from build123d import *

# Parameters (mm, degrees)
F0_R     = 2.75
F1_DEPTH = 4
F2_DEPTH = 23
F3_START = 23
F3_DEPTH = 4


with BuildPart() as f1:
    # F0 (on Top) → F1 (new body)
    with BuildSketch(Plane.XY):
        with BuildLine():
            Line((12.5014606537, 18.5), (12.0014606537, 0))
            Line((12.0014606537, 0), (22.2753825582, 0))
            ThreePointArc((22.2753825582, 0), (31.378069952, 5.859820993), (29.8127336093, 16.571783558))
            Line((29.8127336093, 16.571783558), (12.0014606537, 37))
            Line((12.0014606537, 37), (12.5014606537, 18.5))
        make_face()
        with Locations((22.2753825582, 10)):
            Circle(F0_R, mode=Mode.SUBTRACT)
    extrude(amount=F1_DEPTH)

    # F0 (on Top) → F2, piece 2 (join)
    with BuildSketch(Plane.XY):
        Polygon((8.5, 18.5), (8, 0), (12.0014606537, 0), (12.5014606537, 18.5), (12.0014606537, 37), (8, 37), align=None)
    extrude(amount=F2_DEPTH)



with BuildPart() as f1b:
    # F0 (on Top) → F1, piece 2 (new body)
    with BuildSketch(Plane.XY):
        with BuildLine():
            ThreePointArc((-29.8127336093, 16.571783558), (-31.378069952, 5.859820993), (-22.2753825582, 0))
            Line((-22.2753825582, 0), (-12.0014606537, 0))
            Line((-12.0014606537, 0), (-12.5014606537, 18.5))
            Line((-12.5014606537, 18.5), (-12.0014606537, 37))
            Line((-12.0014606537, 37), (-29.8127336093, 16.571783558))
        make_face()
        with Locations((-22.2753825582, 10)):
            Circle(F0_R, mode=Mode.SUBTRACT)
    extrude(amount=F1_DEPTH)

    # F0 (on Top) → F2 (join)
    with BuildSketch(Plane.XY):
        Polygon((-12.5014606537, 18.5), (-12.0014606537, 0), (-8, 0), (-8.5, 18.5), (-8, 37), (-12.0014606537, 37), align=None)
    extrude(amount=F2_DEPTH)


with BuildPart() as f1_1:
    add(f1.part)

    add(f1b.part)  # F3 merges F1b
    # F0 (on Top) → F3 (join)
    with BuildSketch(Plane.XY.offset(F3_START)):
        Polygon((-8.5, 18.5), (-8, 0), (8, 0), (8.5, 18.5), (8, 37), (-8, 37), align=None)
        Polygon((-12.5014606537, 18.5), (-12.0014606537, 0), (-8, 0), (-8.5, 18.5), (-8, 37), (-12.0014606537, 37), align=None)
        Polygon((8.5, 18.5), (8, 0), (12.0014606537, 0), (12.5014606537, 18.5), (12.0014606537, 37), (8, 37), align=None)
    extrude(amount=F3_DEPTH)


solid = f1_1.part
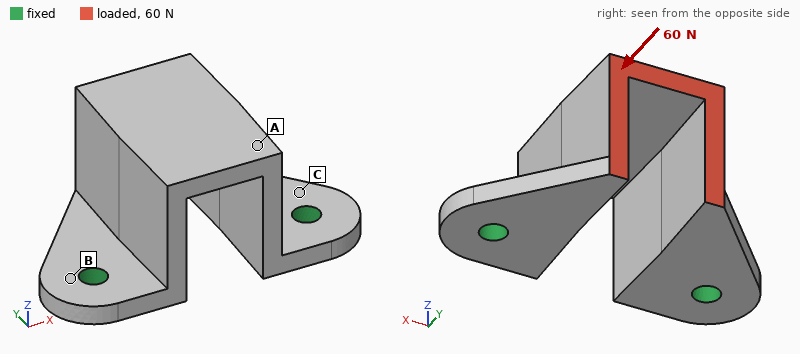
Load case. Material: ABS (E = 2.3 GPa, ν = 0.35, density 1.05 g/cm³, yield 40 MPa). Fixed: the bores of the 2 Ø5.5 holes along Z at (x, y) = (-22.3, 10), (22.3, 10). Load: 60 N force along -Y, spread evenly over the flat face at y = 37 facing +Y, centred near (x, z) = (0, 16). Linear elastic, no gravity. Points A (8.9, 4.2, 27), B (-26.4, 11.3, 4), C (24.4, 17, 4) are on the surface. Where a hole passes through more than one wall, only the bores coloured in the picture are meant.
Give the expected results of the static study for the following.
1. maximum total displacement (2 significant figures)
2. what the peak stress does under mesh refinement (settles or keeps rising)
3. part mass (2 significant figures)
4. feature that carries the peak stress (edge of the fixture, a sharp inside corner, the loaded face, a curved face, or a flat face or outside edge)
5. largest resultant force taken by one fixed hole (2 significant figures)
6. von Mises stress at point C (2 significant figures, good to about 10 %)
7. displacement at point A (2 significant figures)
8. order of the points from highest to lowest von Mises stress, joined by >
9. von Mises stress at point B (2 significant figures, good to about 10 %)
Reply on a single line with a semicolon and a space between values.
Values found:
0.31 mm; keeps rising; 15 g; edge of the fixture; 30 N; 3.0 MPa; 0.23 mm; C > B > A; 1.5 MPa
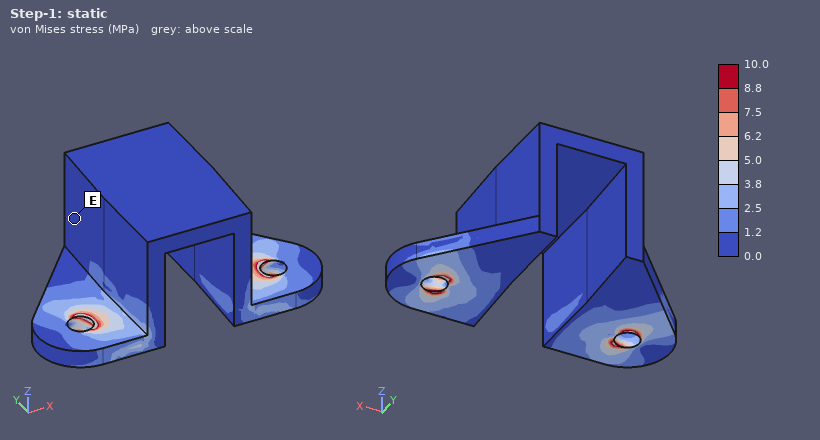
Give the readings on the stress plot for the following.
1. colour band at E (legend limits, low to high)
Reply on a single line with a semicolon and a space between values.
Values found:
0.0 to 1.2 MPa
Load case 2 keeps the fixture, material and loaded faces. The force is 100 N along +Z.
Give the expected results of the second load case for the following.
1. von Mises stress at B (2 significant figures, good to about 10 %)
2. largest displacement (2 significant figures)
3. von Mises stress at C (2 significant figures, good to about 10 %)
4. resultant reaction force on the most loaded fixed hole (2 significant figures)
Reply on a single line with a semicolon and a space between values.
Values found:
4.5 MPa; 0.94 mm; 11 MPa; 54 N
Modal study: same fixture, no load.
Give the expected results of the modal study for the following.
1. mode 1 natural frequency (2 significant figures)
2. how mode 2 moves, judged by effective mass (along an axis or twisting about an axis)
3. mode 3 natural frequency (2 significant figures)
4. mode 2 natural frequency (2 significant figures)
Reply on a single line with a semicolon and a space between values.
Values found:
710 Hz; along X; 1900 Hz; 1400 Hz
